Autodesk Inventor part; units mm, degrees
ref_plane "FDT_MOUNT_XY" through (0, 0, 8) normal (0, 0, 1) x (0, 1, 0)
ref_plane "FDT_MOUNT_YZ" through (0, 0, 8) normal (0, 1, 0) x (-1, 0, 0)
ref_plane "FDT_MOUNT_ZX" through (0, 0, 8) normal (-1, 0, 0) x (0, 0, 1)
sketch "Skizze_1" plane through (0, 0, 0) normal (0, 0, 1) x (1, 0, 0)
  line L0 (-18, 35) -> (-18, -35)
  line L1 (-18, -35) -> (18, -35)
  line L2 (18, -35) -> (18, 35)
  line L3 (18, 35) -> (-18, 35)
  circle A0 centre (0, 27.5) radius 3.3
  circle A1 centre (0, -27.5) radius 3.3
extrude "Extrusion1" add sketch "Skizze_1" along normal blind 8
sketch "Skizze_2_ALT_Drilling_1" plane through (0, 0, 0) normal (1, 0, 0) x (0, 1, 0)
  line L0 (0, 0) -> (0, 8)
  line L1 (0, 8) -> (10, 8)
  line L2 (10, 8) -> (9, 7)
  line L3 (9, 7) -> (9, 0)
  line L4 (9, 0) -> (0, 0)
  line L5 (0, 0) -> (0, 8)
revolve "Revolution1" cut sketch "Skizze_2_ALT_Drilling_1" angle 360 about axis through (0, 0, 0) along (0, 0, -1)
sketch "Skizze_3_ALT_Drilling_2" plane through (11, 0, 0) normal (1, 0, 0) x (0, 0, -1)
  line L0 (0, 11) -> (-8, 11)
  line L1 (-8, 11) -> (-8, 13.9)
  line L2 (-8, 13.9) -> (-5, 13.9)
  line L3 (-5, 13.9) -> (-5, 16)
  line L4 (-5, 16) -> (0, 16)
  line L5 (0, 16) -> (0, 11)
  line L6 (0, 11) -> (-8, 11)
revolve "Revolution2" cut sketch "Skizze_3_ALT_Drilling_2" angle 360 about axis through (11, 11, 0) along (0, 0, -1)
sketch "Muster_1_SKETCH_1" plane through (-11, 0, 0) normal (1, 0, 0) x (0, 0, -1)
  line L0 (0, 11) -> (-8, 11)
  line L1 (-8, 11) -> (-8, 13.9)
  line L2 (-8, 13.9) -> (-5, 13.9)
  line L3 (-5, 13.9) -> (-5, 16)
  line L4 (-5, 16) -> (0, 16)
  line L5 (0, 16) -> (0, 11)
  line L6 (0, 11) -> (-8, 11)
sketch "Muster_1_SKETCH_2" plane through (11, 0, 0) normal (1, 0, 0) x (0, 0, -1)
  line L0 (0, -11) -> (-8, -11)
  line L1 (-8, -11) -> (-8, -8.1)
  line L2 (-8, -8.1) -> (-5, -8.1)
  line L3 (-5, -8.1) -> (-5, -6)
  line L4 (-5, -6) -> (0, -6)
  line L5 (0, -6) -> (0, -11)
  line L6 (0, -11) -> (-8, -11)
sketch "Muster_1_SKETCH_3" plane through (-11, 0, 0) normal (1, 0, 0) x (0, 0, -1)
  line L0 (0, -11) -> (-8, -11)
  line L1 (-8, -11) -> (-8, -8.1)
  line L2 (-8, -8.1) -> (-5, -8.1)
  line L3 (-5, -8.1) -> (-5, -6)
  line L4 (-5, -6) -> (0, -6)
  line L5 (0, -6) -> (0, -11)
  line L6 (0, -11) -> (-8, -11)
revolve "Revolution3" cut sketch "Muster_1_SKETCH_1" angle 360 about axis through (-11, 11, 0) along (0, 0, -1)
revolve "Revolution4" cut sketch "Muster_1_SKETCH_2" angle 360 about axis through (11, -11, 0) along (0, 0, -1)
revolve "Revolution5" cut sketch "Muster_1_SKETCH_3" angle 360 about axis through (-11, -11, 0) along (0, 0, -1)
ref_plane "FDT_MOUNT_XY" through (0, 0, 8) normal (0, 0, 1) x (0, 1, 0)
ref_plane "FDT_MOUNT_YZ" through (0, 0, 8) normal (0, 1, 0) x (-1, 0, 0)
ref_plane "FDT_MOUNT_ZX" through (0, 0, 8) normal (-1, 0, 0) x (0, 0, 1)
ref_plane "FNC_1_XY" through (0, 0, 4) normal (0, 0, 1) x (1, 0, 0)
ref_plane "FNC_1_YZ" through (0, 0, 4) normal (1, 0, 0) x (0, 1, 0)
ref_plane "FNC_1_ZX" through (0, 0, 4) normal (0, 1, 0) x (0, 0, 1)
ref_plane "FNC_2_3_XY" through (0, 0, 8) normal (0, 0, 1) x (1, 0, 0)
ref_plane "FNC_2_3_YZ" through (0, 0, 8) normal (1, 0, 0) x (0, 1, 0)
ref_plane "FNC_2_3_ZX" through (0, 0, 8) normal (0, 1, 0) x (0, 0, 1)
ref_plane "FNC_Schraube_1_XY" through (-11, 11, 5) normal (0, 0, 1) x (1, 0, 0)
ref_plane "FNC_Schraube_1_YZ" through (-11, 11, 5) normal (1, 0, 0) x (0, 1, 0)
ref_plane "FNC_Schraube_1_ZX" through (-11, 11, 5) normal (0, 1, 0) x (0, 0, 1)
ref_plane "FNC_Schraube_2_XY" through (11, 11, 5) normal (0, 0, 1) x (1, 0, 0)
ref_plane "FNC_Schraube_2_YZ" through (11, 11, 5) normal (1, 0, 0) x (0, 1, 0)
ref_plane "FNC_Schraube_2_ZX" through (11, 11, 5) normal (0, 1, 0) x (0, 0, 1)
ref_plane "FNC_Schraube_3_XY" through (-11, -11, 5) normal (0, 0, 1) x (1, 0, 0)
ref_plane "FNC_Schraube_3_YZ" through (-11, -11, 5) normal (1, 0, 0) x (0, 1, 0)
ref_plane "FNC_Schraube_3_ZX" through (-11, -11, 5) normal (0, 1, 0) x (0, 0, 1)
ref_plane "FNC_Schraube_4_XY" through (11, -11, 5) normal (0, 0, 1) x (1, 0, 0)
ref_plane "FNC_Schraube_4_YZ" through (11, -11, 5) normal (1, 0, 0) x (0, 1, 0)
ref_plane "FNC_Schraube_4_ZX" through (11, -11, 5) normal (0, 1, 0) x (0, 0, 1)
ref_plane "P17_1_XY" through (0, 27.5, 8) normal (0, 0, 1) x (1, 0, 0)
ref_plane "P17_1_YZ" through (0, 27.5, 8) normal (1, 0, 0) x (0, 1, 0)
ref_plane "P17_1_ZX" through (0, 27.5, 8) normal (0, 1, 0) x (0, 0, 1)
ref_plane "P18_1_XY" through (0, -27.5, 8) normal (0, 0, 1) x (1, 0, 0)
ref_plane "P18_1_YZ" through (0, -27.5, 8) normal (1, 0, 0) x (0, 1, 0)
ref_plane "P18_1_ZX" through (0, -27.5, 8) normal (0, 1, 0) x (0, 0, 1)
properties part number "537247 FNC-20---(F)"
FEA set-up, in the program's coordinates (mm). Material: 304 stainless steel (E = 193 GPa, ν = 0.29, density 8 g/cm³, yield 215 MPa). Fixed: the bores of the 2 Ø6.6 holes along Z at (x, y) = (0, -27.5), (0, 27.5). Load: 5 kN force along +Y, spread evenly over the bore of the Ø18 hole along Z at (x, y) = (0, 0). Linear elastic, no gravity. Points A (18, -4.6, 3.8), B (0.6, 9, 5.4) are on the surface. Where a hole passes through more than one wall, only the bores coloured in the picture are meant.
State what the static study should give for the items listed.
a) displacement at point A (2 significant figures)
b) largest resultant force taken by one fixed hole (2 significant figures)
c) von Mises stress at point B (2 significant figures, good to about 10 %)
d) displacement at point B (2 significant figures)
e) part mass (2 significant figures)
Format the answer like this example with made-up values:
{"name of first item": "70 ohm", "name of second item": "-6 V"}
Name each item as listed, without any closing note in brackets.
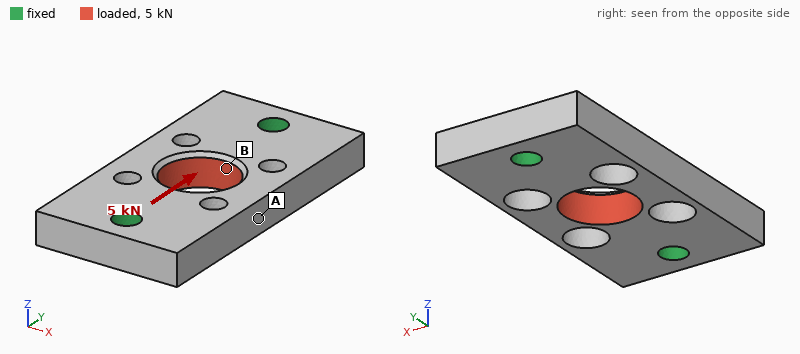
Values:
{"displacement at point A": "1.9 µm", "largest resultant force taken by one fixed hole": "2.5 kN", "von Mises stress at point B": "23 MPa", "displacement at point B": "1.6 µm", "part mass": "130 g"}
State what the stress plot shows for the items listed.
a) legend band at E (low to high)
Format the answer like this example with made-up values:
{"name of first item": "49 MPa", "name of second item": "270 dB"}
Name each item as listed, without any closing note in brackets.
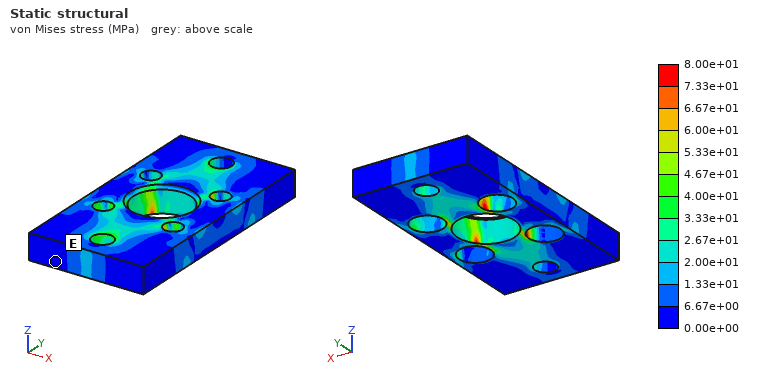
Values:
{"legend band at E": "0.00e+00 to 6.67e+00 MPa"}
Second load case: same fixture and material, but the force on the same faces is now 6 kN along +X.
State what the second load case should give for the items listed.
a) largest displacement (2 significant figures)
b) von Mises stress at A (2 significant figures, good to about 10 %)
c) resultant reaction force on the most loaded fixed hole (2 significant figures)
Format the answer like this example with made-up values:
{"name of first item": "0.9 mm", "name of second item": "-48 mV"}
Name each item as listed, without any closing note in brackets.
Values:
{"largest displacement": "11 µm", "von Mises stress at A": "56 MPa", "resultant reaction force on the most loaded fixed hole": "3.0 kN"}
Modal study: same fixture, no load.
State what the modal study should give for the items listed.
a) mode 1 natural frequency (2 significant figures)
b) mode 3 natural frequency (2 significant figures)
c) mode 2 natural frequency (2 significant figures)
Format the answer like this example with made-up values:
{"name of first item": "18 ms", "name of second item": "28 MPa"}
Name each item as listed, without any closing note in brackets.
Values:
{"mode 1 natural frequency": "11 kHz", "mode 3 natural frequency": "18 kHz", "mode 2 natural frequency": "11 kHz"}
